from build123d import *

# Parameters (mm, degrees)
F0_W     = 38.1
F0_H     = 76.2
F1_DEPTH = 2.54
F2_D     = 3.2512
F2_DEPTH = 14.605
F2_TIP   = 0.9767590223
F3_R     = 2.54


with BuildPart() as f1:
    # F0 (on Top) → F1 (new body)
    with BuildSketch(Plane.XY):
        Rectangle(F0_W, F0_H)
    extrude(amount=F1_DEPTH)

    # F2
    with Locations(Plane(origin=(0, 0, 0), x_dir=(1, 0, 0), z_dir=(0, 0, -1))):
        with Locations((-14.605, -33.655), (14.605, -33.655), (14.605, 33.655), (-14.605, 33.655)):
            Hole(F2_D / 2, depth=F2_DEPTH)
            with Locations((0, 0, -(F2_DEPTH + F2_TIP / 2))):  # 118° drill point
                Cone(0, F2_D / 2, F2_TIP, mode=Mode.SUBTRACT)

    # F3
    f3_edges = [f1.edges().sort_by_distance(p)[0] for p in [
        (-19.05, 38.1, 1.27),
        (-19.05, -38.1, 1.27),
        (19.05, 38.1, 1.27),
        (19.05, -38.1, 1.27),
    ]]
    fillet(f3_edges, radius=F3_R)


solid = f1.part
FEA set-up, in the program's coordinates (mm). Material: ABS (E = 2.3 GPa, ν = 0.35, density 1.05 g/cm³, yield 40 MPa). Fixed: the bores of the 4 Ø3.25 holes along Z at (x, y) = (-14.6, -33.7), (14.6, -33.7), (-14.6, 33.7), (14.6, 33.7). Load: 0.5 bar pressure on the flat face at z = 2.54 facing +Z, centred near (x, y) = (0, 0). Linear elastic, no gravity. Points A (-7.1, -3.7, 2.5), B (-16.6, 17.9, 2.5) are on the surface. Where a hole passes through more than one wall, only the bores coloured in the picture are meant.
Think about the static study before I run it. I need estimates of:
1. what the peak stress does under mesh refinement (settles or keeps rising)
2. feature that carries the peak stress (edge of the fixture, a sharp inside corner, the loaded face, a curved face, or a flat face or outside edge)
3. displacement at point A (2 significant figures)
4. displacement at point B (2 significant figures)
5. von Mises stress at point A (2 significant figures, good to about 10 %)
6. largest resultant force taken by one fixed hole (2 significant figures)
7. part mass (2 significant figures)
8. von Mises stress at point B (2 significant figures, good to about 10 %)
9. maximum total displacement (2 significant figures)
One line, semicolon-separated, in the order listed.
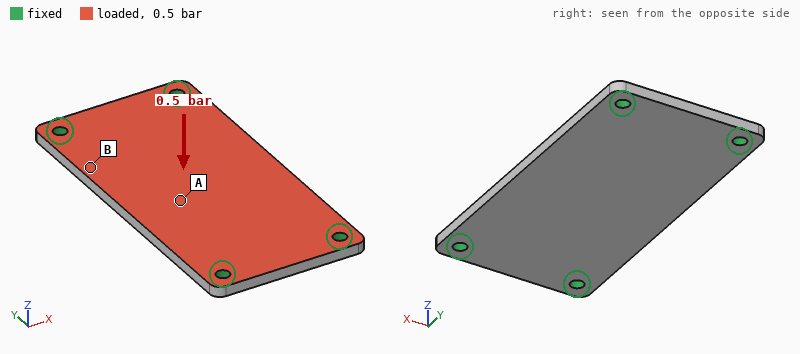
keeps rising; edge of the fixture; 0.91 mm; 0.49 mm; 8.1 MPa; 36 N; 7.6 g; 3.5 MPa; 0.98 mm
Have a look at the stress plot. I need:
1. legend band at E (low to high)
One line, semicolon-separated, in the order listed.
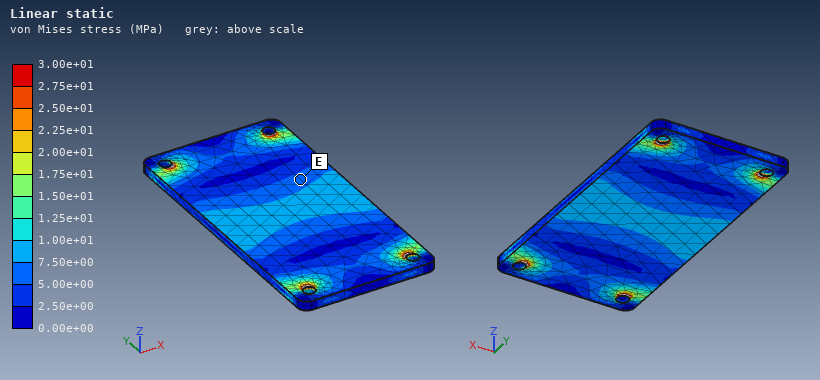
5.00e+00 to 7.50e+00 MPa
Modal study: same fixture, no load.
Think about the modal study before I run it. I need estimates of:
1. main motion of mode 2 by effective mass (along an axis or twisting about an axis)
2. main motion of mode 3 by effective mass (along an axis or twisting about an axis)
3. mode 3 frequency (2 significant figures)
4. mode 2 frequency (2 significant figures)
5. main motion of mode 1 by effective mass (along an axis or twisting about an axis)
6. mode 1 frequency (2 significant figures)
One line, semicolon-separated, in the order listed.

twisting about Y; twisting about X; 2200 Hz; 1300 Hz; along Z; 810 Hz
